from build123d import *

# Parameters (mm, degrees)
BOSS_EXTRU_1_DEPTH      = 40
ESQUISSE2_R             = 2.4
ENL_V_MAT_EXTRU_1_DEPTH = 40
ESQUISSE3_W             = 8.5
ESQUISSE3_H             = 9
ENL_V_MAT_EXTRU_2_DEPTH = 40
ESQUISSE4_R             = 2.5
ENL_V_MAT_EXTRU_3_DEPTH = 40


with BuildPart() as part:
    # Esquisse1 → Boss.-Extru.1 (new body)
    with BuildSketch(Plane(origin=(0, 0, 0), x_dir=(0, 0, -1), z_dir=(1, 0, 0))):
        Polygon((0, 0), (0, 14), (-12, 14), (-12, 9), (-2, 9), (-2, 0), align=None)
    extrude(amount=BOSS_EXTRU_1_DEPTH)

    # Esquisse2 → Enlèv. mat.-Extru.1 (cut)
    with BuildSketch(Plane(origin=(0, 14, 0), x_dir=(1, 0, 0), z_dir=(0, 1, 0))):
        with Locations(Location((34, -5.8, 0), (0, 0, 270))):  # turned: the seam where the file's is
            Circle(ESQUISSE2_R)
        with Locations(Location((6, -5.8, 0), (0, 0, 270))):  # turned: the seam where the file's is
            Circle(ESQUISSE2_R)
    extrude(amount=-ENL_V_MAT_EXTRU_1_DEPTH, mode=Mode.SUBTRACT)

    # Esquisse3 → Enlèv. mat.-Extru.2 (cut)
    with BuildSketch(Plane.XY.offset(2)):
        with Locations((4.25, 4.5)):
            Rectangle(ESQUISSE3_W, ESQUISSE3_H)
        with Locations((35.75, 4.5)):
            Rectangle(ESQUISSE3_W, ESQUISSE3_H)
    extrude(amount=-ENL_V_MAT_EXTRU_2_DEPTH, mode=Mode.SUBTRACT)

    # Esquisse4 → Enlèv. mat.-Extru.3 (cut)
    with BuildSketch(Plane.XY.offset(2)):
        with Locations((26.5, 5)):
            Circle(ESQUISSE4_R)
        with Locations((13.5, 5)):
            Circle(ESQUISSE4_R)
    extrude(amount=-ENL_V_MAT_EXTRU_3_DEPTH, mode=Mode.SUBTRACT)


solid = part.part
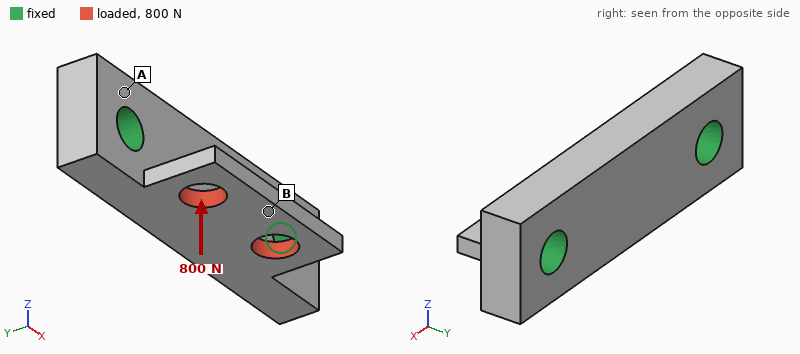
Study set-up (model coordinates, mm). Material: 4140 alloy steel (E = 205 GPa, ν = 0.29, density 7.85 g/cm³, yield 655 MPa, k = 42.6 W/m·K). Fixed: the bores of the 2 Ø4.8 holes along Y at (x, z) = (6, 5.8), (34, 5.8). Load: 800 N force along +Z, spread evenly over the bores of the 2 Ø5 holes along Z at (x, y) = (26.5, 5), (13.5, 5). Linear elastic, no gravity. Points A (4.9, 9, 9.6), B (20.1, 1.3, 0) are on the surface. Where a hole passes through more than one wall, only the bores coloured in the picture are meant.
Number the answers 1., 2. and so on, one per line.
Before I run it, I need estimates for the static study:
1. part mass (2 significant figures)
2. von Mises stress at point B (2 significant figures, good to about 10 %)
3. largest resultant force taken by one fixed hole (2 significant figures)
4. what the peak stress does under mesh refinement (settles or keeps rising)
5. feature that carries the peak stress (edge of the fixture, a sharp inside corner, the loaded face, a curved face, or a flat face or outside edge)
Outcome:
1. 20 g
2. 40 MPa
3. 400 N
4. keeps rising
5. a sharp inside corner
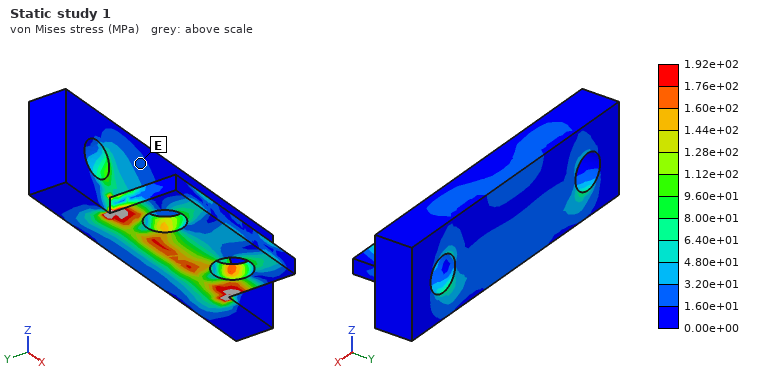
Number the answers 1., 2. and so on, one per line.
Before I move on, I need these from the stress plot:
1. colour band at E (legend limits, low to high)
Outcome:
1. 1.60e+01 to 3.20e+01 MPa
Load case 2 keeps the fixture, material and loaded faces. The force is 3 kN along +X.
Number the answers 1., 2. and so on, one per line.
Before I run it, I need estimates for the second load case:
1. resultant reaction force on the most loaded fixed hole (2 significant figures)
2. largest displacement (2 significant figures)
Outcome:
1. 1.8 kN
2. 15 µm
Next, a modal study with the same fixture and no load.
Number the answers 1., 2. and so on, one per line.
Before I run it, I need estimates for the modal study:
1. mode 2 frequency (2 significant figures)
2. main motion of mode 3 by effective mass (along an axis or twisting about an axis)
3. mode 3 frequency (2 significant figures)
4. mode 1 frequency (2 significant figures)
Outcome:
1. 20 kHz
2. along Y
3. 33 kHz
4. 14 kHz
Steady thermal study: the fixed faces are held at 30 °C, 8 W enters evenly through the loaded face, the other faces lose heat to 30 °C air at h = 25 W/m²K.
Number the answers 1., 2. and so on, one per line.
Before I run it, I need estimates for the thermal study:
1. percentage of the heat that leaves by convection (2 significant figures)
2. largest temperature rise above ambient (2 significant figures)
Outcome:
1. 5.9 %
2. 44 K
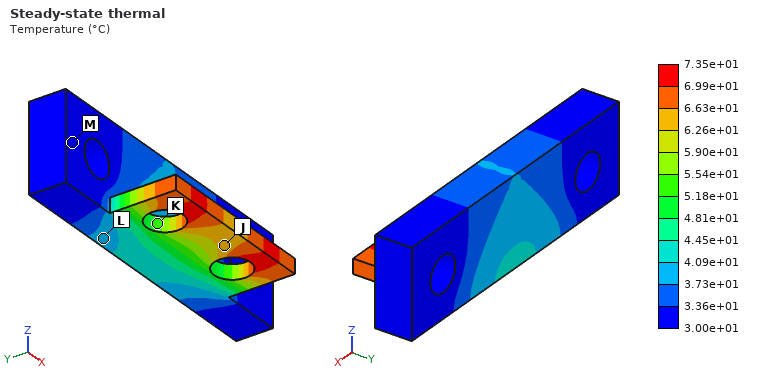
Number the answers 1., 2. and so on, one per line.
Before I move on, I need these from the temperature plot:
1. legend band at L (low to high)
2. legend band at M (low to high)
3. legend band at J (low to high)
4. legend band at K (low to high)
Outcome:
1. 3.73e+01 to 4.09e+01 °C
2. 3.00e+01 to 3.36e+01 °C
3. 6.26e+01 to 6.63e+01 °C
4. 5.18e+01 to 5.54e+01 °C
